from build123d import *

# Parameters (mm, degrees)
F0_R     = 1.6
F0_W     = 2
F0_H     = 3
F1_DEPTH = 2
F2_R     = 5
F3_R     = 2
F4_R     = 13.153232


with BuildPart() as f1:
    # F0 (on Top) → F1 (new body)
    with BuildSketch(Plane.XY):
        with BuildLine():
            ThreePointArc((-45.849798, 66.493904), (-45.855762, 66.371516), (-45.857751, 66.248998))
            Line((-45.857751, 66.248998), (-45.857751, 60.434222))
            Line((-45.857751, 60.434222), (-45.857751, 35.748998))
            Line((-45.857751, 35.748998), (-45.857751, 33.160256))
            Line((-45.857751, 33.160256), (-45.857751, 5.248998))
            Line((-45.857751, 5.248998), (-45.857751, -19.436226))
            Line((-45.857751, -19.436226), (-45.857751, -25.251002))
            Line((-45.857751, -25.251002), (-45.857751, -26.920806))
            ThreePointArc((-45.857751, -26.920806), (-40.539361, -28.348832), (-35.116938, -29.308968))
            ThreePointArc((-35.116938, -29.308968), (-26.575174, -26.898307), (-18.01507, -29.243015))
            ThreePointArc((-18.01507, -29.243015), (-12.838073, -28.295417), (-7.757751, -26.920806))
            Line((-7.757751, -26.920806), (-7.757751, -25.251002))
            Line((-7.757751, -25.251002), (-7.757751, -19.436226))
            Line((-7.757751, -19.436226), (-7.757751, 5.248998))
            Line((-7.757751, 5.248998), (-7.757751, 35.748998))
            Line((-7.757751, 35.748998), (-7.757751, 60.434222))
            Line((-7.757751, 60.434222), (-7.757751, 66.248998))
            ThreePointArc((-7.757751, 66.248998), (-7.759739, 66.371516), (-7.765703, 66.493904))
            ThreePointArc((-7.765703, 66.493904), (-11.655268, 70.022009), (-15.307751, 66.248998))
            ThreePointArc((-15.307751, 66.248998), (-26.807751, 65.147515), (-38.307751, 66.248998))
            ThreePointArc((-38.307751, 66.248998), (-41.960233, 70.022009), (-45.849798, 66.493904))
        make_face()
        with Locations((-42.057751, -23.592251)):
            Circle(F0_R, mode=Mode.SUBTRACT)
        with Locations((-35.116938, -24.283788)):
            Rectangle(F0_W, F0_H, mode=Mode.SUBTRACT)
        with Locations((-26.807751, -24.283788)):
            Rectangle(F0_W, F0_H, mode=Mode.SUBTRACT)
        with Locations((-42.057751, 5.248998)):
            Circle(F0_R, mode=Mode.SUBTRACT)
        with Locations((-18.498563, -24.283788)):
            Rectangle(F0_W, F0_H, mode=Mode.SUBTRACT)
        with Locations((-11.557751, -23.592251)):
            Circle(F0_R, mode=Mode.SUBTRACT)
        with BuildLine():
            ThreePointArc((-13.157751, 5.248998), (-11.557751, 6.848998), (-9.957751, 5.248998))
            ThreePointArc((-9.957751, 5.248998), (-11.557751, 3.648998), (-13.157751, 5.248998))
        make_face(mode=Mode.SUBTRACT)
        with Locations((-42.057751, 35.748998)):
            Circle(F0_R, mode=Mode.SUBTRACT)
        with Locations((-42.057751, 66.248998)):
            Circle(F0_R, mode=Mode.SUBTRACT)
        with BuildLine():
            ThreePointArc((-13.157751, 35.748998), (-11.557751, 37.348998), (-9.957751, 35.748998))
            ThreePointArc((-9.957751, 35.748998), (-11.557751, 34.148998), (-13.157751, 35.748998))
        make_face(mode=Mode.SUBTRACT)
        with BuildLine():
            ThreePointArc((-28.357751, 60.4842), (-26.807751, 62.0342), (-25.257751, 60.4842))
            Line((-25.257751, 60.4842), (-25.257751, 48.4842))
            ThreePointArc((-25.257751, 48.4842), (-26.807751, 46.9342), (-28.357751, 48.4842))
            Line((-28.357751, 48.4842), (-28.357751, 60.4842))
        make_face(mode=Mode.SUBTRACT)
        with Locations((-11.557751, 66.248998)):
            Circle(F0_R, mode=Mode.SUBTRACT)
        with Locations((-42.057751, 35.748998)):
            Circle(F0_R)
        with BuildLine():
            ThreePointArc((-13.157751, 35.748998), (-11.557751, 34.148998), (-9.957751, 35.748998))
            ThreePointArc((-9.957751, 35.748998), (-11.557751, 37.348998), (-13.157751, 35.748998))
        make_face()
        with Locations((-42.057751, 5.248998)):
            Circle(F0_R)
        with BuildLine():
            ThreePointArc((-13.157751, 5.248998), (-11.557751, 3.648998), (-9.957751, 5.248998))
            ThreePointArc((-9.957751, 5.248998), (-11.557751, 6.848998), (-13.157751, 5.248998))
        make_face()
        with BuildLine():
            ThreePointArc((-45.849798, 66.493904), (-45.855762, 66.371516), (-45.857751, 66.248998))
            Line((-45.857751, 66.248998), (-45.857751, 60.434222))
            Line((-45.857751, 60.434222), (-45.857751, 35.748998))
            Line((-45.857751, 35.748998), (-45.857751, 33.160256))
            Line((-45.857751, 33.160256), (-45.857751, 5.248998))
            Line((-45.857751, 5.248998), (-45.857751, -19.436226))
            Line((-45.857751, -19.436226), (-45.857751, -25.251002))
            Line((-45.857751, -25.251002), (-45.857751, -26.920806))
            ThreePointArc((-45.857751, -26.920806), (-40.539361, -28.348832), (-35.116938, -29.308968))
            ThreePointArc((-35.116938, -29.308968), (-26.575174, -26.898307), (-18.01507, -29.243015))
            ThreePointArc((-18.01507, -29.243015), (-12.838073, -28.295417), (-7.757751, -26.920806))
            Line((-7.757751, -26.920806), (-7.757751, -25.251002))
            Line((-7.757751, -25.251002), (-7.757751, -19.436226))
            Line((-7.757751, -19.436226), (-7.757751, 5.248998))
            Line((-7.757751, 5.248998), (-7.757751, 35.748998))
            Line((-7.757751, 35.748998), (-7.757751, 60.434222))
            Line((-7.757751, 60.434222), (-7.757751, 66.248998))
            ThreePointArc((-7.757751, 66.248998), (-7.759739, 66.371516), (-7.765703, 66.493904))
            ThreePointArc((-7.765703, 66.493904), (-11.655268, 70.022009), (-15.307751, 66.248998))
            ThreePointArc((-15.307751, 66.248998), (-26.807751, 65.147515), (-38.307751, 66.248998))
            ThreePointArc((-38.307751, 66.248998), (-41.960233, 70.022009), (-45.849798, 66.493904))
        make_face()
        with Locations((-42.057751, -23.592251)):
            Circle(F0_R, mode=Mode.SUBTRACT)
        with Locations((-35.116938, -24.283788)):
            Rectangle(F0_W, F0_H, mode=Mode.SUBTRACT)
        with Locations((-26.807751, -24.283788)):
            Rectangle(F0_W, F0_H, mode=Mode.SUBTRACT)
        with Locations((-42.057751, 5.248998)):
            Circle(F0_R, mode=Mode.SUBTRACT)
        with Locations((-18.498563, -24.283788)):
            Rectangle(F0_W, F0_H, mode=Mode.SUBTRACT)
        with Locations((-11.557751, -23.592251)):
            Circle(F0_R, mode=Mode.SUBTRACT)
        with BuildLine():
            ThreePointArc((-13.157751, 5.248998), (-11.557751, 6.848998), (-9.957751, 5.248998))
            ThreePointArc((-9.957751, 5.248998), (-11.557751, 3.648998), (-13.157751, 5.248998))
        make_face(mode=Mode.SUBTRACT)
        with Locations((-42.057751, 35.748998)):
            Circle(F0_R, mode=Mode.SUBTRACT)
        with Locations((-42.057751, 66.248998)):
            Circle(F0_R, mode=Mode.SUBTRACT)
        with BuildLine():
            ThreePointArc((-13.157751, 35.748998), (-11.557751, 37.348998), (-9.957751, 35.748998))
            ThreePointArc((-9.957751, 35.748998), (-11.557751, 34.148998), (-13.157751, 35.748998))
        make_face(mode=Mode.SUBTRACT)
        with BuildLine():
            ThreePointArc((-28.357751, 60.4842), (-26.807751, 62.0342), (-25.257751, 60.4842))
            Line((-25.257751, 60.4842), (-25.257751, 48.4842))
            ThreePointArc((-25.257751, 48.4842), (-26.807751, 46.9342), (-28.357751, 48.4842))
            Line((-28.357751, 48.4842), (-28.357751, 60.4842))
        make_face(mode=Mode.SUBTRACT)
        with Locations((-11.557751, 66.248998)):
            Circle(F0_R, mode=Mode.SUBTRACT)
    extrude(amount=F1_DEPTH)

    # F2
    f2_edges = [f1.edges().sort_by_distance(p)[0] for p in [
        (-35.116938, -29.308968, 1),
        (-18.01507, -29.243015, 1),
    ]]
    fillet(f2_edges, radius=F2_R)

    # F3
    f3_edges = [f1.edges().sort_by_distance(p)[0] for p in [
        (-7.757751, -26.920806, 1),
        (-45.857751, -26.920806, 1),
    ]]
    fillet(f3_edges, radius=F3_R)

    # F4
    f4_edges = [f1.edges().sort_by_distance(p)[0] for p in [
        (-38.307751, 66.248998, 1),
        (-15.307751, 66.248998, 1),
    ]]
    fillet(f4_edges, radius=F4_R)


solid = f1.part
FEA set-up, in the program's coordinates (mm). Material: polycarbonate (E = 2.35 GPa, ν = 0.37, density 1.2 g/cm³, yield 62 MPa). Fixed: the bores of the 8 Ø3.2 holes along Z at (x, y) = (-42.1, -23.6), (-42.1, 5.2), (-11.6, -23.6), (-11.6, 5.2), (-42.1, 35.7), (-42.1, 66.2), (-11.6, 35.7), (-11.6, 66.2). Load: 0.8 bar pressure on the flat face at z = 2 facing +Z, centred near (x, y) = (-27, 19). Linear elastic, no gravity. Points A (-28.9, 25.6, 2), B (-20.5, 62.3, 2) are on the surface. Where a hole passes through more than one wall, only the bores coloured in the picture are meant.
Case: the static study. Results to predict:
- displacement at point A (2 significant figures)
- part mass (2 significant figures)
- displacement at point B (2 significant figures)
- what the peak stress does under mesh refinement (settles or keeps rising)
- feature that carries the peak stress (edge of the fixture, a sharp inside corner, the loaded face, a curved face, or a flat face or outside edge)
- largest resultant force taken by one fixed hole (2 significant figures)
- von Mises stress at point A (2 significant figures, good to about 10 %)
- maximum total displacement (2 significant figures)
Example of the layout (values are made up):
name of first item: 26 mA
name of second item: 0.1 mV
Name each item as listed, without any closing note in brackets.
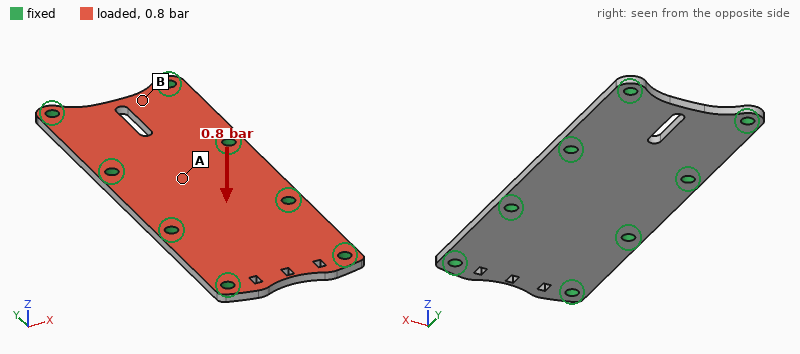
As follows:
displacement at point A: 0.20 mm
part mass: 8.4 g
displacement at point B: 0.14 mm
what the peak stress does under mesh refinement: keeps rising
feature that carries the peak stress: edge of the fixture
largest resultant force taken by one fixed hole: 46 N
von Mises stress at point A: 4.3 MPa
maximum total displacement: 0.30 mm
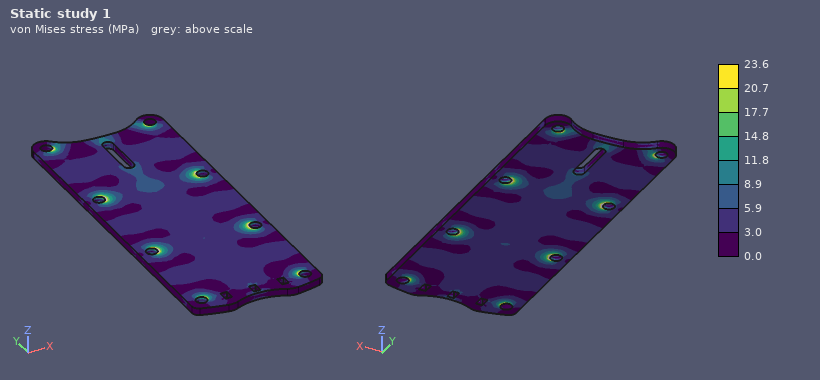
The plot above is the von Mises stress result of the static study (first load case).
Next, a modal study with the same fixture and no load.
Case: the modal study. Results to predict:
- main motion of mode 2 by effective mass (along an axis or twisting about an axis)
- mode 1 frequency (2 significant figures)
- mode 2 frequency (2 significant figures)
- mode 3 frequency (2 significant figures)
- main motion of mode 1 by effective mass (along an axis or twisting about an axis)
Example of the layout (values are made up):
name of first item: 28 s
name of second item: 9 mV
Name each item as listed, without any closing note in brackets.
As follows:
main motion of mode 2 by effective mass: along Z
mode 1 frequency: 2200 Hz
mode 2 frequency: 2400 Hz
mode 3 frequency: 2500 Hz
main motion of mode 1 by effective mass: along Z
